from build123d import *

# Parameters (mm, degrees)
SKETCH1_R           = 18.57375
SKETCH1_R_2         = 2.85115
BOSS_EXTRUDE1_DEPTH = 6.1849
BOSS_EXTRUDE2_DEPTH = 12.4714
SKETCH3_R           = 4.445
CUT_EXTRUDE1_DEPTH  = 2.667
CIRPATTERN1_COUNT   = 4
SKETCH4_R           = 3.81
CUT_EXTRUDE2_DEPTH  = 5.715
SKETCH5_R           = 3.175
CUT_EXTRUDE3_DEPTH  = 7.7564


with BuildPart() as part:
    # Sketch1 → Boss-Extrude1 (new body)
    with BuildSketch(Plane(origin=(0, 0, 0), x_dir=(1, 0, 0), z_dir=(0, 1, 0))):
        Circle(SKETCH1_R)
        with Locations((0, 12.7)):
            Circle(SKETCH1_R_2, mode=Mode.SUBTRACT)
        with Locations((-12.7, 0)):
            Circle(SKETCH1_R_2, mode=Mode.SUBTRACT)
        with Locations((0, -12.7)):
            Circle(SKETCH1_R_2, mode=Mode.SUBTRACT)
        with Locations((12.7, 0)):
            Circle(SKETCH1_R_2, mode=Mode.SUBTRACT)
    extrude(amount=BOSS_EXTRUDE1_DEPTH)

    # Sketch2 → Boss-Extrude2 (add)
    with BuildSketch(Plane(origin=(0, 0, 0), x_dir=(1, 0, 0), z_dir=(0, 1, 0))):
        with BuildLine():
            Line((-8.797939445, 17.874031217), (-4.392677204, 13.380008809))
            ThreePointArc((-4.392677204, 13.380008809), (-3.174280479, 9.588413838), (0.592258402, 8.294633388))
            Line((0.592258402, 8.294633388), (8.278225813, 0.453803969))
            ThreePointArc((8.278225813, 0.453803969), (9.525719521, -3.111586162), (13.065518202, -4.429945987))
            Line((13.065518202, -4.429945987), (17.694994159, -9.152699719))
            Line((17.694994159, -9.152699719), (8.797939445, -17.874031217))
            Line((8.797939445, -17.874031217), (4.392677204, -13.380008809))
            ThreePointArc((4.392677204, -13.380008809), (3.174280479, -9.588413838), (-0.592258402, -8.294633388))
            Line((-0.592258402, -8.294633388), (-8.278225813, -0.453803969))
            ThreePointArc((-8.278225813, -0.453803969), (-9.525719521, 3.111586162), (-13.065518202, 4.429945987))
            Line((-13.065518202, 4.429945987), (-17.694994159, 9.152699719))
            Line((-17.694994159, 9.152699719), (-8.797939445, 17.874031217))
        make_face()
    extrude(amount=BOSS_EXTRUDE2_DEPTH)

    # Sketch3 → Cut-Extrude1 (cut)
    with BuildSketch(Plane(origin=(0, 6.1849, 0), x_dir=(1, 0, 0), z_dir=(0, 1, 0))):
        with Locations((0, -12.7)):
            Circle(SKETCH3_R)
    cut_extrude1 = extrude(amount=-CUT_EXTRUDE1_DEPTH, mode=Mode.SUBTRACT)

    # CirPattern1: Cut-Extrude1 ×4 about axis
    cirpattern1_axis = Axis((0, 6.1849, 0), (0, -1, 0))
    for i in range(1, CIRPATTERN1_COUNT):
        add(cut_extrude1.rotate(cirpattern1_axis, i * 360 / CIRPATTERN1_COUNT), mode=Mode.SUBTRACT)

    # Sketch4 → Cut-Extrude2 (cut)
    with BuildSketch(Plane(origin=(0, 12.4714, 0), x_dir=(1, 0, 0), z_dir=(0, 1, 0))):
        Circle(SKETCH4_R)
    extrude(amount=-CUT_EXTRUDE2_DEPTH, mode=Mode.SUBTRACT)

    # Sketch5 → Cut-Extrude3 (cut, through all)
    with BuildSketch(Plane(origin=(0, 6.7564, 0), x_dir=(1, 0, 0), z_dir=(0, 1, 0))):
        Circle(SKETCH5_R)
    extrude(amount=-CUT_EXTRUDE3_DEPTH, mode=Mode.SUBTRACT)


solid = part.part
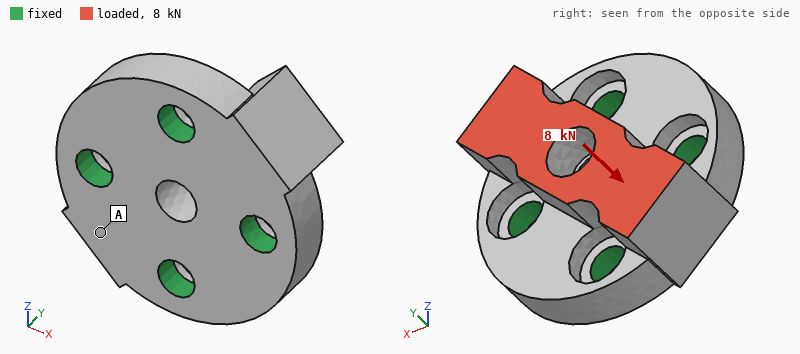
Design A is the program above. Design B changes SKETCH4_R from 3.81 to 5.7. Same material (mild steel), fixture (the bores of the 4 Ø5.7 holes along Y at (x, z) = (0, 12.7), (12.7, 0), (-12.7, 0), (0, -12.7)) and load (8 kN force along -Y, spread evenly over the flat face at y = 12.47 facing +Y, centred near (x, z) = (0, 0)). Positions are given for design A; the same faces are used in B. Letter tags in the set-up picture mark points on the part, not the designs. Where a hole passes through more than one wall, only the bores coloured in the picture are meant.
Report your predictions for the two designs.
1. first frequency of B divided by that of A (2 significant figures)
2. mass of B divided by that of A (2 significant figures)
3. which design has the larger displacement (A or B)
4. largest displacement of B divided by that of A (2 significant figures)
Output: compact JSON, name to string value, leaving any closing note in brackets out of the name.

{"first frequency of B divided by that of A": "0.97", "mass of B divided by that of A": "0.96", "which design has the larger displacement": "B", "largest displacement of B divided by that of A": "1.4"}
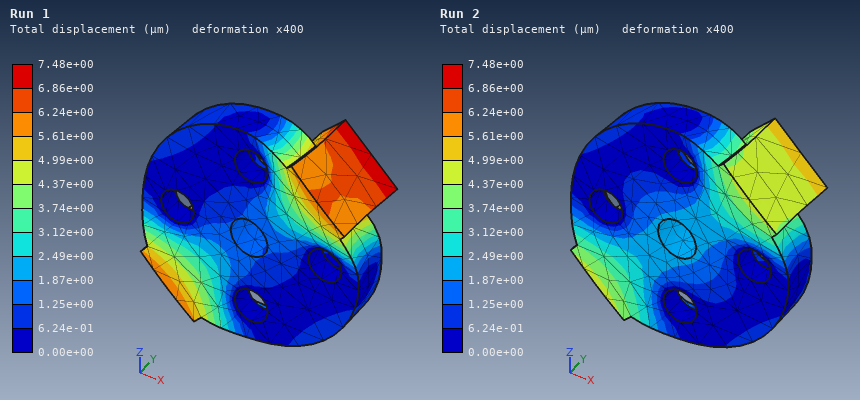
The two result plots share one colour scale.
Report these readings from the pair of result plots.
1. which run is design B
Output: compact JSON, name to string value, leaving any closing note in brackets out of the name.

{"which run is design B": "Run 1"}
